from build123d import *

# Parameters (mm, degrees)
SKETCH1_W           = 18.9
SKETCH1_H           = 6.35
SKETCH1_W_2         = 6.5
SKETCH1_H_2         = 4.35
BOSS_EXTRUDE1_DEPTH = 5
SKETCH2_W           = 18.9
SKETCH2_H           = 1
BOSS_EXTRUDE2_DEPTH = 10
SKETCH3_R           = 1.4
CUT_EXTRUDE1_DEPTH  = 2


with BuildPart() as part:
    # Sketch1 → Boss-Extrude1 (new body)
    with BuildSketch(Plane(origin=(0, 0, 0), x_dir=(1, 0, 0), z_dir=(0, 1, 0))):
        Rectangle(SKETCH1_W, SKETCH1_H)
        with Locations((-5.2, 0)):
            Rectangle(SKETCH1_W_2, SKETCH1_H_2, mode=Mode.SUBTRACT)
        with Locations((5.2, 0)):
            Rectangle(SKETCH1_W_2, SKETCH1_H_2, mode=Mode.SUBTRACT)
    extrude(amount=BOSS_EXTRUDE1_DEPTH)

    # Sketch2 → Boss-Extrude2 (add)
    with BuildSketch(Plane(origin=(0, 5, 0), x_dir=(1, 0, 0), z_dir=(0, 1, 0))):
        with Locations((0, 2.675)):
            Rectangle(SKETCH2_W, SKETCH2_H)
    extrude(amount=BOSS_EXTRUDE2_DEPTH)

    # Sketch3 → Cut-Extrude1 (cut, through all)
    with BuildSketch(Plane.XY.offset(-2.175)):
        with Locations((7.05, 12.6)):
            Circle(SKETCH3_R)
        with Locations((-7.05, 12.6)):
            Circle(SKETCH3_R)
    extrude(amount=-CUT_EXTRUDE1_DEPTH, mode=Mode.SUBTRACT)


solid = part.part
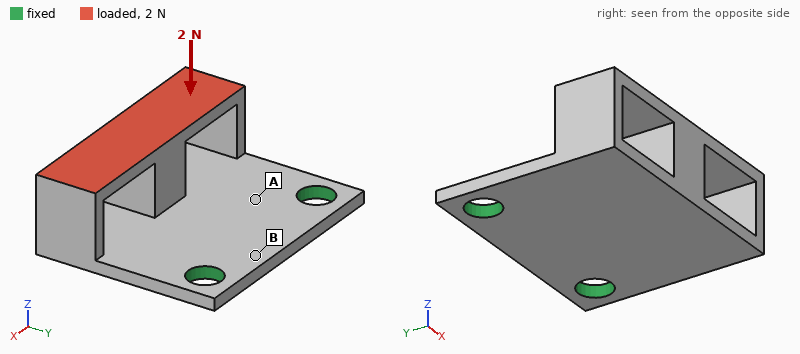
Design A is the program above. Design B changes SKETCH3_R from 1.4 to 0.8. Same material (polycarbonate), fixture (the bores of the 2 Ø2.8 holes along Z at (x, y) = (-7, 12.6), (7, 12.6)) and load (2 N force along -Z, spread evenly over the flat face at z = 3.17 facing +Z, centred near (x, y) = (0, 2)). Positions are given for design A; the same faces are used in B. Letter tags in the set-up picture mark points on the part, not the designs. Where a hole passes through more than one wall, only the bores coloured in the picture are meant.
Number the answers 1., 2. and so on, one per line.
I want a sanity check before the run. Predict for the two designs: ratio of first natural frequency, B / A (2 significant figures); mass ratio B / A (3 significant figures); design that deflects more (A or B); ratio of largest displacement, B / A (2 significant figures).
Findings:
1. 0.88
2. 1.02
3. B
4. 1.3
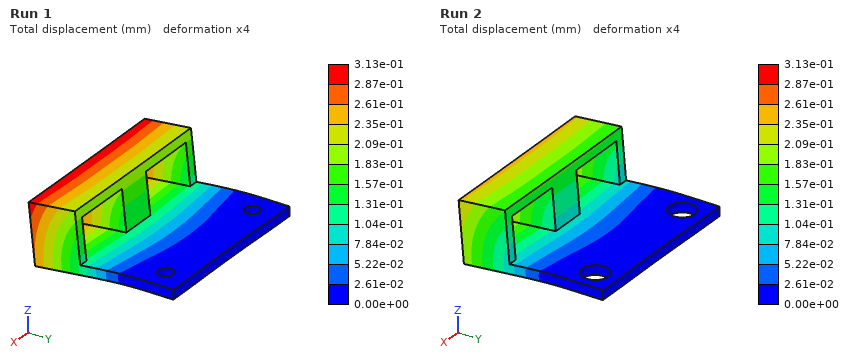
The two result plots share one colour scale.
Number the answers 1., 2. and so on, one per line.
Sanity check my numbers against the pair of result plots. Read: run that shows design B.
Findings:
1. Run 1
